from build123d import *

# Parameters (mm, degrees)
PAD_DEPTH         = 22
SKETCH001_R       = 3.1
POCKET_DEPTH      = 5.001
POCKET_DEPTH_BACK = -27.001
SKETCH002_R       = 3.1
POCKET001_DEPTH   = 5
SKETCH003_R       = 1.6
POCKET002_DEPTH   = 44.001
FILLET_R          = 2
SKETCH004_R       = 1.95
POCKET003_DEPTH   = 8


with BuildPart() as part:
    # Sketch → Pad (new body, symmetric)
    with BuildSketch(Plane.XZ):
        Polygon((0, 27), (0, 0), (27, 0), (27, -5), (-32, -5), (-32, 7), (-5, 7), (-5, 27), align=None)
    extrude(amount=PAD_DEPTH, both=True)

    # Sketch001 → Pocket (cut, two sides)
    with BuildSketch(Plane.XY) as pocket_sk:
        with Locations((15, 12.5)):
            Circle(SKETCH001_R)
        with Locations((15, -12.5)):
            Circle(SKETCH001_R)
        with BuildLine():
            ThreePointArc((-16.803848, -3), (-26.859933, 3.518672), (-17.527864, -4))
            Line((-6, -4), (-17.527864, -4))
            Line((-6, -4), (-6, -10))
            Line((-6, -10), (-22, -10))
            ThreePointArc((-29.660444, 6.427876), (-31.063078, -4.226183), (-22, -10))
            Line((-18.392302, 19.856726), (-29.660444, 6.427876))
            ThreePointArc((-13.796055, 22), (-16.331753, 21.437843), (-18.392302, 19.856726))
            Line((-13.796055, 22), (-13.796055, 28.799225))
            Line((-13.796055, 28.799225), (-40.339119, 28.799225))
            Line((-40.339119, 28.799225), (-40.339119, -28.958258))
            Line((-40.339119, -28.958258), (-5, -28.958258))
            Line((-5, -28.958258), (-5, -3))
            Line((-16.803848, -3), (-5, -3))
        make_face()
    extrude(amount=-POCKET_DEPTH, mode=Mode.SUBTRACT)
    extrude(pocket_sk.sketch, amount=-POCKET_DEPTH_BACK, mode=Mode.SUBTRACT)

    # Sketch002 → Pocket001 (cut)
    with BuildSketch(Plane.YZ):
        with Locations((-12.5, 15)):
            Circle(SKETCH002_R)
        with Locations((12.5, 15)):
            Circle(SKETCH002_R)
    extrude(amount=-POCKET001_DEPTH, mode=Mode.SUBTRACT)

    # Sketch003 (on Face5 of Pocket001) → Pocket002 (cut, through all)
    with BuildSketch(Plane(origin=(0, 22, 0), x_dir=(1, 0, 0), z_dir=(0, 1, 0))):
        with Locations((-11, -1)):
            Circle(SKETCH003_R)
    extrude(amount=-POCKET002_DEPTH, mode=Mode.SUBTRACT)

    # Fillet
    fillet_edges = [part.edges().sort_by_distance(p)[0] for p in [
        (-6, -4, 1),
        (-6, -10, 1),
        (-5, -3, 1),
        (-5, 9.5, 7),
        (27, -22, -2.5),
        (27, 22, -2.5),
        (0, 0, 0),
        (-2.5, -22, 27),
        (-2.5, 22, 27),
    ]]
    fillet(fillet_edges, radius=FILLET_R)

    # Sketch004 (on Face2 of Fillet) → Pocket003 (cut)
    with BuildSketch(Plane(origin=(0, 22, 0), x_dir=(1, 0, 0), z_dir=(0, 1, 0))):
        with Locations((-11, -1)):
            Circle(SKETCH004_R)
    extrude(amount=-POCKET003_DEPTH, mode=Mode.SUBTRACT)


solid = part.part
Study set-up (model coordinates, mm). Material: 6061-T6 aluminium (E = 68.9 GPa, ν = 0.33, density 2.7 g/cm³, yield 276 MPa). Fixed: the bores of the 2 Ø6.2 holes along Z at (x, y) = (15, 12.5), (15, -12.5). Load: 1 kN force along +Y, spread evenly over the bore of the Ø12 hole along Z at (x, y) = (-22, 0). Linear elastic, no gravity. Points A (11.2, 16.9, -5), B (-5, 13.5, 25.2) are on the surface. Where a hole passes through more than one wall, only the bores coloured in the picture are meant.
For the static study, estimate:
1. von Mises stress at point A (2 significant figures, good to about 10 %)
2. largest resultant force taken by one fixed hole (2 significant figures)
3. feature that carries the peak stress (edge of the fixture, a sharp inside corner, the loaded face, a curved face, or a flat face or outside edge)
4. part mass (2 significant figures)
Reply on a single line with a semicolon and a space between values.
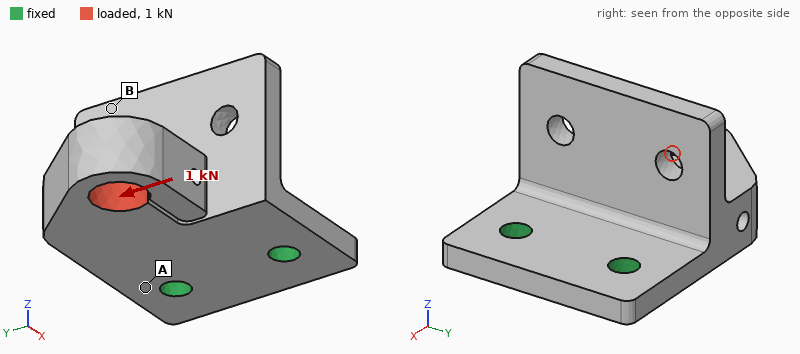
25 MPa; 1.5 kN; the loaded face; 51 g
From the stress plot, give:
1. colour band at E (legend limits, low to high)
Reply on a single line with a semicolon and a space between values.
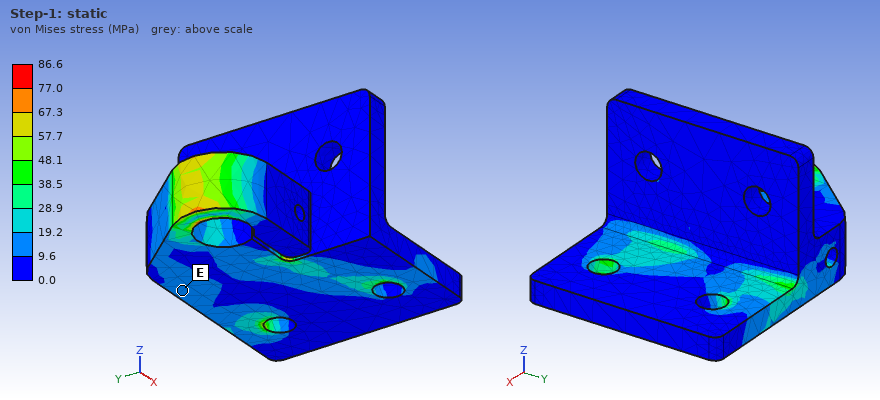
9.6 to 19.2 MPa
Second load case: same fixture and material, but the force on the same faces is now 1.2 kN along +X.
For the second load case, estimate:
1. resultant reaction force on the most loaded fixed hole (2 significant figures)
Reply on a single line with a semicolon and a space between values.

640 N
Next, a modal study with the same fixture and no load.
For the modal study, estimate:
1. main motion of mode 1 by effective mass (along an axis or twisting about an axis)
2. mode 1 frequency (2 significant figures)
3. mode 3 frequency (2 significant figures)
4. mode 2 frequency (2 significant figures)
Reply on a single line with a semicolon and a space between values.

along Z; 1700 Hz; 3200 Hz; 2500 Hz
